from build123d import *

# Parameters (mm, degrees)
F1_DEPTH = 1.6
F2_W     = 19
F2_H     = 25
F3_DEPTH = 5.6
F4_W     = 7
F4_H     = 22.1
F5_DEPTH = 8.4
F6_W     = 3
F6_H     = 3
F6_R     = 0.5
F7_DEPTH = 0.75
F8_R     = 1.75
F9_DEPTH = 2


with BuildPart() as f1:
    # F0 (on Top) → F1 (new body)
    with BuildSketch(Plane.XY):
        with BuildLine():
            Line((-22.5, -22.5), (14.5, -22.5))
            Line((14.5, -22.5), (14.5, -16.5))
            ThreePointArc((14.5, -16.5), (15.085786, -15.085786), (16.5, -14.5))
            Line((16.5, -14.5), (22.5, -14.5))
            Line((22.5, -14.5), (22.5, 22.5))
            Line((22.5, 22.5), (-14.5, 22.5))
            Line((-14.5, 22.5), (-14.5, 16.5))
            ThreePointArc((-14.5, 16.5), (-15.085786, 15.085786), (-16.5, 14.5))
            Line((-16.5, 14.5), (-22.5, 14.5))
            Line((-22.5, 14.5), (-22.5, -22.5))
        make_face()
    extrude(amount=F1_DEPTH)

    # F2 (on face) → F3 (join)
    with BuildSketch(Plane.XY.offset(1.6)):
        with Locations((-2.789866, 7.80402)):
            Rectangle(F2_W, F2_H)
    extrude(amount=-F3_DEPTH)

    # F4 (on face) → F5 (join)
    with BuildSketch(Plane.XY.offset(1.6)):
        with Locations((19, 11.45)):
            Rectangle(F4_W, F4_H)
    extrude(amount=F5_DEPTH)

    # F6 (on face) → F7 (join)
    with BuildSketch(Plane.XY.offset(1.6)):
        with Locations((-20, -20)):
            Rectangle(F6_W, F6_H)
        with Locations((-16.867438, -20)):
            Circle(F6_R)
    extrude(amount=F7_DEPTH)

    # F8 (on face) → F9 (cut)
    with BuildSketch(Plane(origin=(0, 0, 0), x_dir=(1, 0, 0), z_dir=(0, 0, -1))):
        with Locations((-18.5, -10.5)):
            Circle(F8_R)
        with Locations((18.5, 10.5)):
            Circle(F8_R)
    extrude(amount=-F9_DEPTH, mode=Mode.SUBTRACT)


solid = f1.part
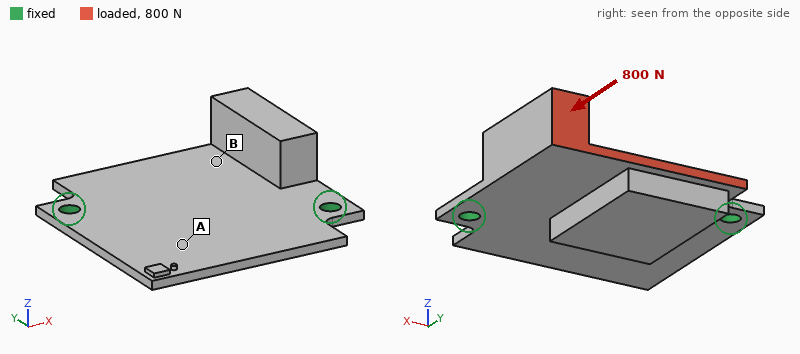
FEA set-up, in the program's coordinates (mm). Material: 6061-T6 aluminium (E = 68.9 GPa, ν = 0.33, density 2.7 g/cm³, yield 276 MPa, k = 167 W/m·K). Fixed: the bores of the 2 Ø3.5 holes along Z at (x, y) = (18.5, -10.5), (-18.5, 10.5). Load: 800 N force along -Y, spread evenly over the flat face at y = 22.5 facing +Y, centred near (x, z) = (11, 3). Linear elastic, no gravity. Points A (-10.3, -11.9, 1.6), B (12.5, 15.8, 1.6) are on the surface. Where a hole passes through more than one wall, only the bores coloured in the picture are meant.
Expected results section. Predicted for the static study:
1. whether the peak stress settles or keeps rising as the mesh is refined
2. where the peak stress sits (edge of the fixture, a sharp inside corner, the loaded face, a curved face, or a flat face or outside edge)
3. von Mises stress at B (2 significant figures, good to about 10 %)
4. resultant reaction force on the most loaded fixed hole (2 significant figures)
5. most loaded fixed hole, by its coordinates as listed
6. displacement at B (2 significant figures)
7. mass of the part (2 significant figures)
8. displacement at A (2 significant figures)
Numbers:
keeps rising
edge of the fixture
45 MPa
650 N
(18.5, -10.5)
0.22 mm
17 g
0.14 mm
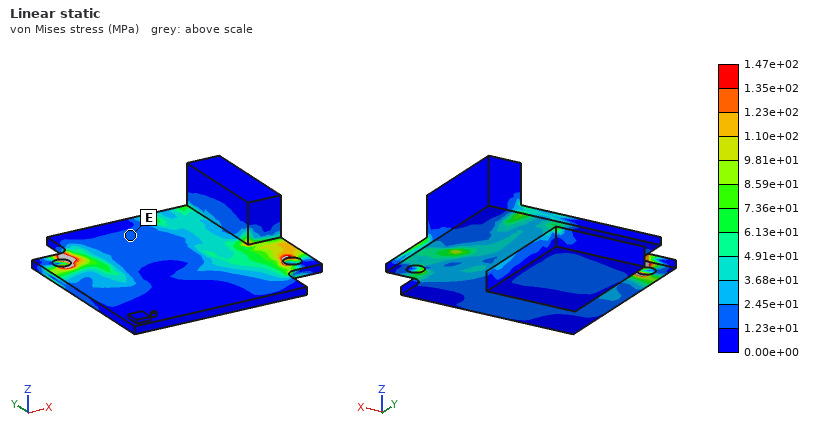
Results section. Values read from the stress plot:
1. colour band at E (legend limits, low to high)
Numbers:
1.23e+01 to 2.45e+01 MPa
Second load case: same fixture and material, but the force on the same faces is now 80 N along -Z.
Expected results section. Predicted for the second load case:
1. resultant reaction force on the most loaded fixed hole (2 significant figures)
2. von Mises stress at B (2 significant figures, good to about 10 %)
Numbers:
71 N
31 MPa
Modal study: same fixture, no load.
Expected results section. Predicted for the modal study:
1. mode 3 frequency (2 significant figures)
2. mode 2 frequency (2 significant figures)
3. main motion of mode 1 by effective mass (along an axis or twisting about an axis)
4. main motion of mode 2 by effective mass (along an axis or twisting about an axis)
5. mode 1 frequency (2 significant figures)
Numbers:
3900 Hz
2800 Hz
along Z
along Z
1200 Hz
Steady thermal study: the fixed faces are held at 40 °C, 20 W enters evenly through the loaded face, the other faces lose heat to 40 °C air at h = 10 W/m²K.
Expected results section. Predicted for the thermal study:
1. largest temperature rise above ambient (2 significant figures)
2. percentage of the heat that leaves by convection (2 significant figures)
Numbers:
48 K
5.0 %
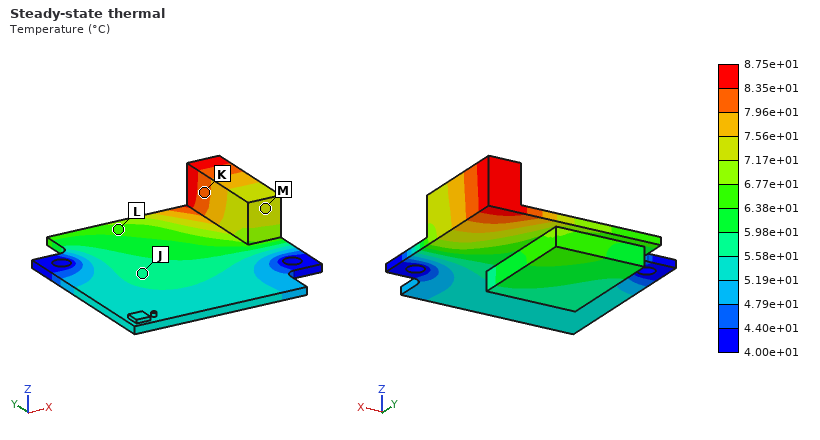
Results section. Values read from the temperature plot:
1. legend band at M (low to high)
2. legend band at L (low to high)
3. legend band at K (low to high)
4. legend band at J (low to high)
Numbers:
7.17e+01 to 7.56e+01 °C
6.38e+01 to 6.77e+01 °C
7.96e+01 to 8.35e+01 °C
5.58e+01 to 5.98e+01 °C
